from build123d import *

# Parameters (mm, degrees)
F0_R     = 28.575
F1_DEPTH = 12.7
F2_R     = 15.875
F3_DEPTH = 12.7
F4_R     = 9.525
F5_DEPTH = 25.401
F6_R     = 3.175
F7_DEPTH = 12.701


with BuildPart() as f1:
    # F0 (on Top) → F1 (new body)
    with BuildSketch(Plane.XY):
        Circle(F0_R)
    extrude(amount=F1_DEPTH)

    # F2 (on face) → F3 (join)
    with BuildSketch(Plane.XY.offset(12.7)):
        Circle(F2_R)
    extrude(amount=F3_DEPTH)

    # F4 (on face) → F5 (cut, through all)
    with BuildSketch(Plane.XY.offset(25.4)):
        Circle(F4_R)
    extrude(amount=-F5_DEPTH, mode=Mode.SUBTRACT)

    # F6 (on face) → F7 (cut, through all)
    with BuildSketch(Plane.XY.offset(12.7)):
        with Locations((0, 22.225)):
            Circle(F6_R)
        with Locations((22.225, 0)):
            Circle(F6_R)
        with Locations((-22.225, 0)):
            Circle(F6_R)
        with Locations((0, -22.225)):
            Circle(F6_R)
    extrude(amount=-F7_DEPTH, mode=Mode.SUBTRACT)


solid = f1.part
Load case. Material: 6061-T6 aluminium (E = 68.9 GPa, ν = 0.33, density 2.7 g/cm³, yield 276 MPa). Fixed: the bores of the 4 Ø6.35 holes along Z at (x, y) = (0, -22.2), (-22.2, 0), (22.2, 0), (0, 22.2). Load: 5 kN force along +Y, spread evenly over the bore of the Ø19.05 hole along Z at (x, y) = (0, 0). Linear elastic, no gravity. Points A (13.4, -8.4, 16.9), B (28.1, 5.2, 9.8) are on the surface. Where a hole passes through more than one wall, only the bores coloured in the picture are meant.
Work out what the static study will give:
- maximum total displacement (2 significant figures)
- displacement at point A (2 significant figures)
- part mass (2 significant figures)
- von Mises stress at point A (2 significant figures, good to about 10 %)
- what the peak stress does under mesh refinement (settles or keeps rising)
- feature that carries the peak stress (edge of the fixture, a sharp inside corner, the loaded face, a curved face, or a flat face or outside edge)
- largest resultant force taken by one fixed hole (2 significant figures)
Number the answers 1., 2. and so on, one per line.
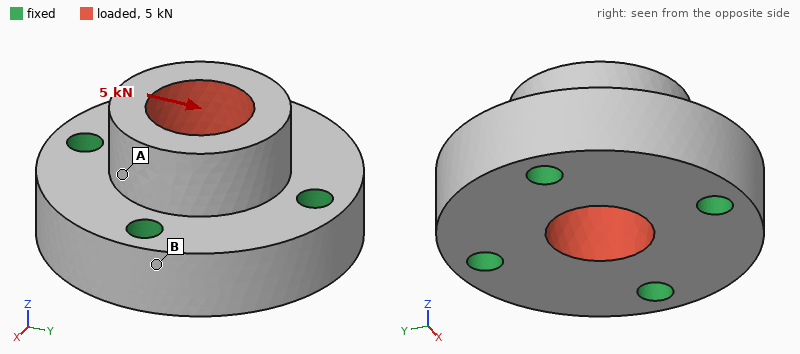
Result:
1. 5.7 µm
2. 2.9 µm
3. 91 g
4. 6.1 MPa
5. keeps rising
6. a sharp inside corner
7. 1.6 kN
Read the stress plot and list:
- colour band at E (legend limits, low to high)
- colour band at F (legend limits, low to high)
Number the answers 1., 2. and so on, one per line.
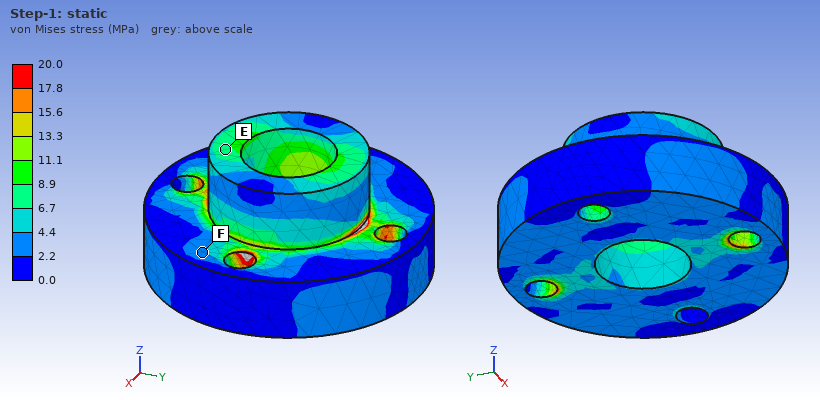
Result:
1. 6.7 to 8.9 MPa
2. 2.2 to 4.4 MPa
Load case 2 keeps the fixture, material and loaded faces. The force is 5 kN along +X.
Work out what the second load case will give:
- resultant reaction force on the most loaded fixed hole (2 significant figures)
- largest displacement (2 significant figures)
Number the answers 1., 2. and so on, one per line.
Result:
1. 1.6 kN
2. 5.7 µm
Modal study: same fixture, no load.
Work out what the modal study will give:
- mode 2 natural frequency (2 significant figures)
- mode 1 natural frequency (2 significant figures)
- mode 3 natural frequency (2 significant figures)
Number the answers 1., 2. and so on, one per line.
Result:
1. 29 kHz
2. 29 kHz
3. 31 kHz
